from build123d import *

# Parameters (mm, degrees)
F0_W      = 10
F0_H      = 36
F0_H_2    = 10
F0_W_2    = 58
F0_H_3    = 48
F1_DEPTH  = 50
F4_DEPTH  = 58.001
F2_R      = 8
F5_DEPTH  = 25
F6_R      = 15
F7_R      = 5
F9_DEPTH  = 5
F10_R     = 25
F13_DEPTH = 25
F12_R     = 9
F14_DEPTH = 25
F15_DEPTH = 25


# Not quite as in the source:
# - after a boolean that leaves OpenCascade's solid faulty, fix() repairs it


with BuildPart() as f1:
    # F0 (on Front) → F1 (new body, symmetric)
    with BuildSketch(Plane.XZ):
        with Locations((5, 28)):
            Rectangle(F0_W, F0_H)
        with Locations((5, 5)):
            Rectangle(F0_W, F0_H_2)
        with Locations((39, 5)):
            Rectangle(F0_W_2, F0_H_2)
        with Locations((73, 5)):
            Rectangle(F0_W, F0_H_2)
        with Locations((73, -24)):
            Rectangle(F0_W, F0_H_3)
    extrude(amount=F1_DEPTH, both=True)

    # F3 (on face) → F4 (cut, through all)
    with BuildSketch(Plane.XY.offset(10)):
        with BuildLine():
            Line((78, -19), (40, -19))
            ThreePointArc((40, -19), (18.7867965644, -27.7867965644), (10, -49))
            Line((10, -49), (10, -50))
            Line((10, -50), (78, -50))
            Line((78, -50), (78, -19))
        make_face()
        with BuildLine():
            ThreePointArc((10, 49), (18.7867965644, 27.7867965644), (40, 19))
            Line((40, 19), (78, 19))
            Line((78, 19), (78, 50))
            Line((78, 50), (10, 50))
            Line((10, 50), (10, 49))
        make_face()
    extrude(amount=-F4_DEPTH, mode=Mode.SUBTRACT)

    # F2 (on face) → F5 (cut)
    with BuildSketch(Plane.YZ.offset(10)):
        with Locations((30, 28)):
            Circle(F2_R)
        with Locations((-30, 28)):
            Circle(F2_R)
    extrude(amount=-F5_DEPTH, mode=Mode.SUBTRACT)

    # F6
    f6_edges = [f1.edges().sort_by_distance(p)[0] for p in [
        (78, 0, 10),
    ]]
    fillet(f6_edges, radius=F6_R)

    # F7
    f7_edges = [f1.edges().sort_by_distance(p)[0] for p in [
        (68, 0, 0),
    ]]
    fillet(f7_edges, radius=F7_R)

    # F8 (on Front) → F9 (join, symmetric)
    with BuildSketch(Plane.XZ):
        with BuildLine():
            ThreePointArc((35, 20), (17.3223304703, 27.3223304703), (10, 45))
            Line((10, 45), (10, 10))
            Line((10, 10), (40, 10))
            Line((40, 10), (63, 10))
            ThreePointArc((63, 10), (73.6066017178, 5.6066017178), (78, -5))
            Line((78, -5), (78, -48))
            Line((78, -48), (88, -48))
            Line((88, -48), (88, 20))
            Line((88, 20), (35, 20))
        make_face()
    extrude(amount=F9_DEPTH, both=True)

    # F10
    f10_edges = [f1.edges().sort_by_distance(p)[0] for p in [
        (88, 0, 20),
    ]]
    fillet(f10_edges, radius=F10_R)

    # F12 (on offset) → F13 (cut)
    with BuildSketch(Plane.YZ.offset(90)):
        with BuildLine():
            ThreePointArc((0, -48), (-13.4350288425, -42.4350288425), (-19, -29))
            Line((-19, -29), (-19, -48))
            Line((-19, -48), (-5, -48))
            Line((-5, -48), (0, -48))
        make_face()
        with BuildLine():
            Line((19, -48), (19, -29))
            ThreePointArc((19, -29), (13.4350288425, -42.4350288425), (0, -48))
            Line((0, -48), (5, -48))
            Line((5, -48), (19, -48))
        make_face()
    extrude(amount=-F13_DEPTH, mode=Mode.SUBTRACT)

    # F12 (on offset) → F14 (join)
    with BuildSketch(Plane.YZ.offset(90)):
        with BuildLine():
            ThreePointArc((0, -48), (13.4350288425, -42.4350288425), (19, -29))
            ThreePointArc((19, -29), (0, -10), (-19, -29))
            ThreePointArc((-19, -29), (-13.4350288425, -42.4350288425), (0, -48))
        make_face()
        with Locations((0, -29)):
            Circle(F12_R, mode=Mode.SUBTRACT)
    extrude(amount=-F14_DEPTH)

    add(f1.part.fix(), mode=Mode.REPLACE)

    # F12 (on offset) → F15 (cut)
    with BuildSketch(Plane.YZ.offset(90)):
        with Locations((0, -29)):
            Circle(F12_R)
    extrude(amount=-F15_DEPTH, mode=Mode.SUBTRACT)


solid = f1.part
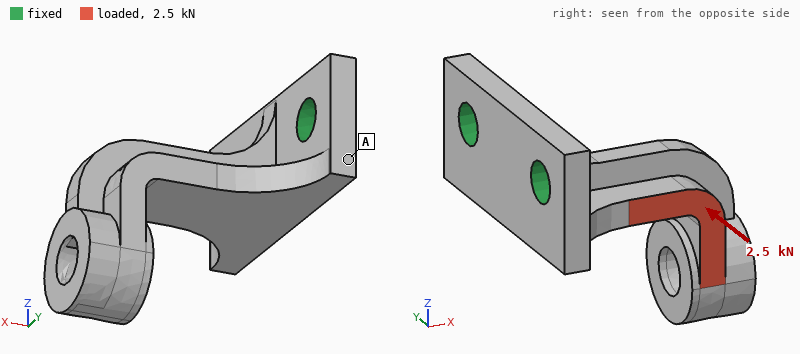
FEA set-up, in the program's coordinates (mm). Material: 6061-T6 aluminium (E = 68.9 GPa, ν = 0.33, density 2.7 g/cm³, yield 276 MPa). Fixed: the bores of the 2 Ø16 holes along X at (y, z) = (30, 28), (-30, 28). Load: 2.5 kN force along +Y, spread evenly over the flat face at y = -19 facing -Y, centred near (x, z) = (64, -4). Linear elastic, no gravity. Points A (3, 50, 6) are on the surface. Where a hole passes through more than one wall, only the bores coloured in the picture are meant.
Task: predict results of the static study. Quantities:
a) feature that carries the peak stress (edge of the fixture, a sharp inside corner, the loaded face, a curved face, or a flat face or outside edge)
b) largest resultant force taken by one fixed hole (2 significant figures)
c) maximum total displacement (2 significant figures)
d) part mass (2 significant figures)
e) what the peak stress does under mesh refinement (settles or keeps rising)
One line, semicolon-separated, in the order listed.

edge of the fixture; 3.0 kN; 0.24 mm; 290 g; keeps rising
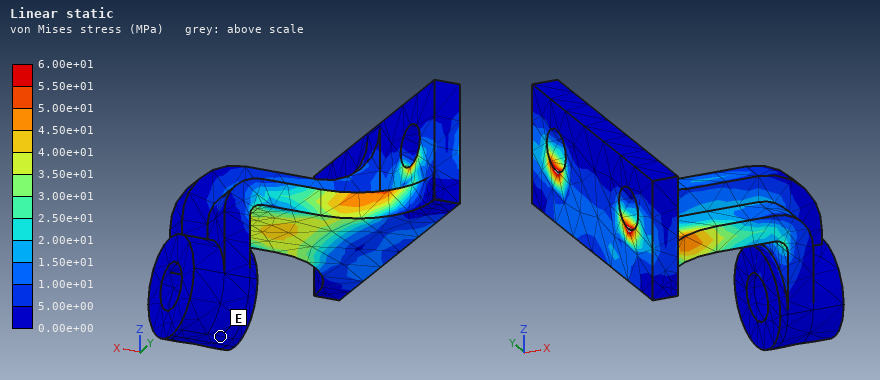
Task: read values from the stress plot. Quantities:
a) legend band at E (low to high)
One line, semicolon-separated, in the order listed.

0.00e+00 to 5.00e+00 MPa
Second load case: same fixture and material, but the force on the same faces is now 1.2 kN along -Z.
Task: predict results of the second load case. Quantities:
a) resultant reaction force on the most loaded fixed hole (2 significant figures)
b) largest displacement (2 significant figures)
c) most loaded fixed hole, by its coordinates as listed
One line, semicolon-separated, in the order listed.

970 N; 0.30 mm; (-30, 28)
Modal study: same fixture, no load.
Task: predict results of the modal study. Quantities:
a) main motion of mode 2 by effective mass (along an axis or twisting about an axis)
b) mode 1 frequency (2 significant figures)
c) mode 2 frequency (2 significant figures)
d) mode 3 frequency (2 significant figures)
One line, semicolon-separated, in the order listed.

along Y; 970 Hz; 1400 Hz; 3100 Hz
